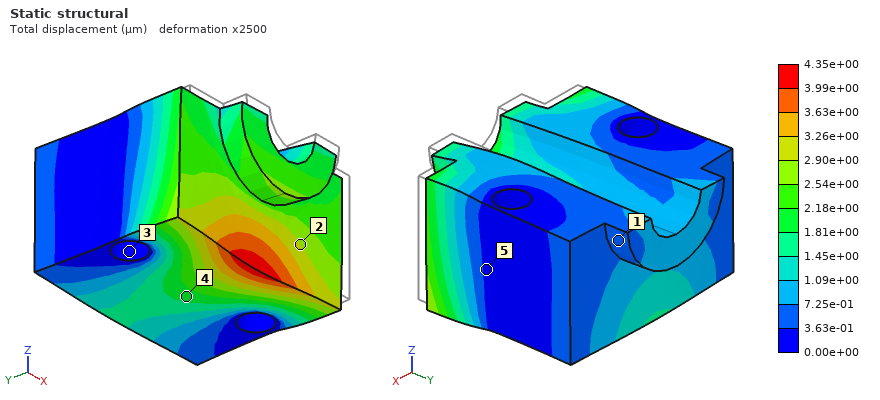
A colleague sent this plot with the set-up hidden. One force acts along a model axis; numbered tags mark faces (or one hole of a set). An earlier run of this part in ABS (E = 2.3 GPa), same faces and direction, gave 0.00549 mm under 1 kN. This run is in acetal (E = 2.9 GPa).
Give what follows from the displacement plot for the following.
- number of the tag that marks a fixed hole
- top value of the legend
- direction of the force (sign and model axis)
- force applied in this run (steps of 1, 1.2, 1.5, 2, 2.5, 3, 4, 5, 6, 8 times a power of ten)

3
4.35e+00 µm
+Y
1 kN
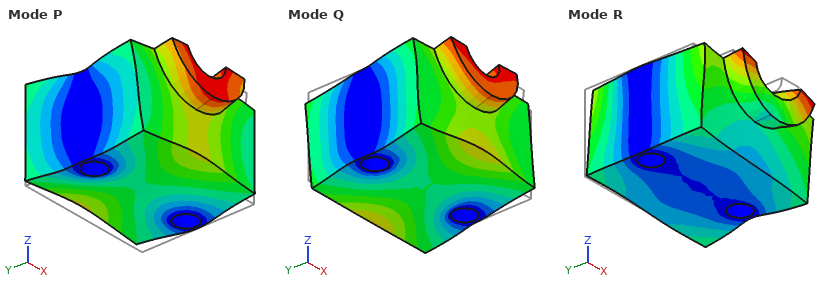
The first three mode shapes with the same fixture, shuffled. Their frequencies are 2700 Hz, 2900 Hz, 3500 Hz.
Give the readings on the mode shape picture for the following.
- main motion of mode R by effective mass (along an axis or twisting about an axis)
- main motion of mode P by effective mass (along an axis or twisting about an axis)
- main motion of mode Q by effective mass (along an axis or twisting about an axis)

along X
along Z
twisting about X
